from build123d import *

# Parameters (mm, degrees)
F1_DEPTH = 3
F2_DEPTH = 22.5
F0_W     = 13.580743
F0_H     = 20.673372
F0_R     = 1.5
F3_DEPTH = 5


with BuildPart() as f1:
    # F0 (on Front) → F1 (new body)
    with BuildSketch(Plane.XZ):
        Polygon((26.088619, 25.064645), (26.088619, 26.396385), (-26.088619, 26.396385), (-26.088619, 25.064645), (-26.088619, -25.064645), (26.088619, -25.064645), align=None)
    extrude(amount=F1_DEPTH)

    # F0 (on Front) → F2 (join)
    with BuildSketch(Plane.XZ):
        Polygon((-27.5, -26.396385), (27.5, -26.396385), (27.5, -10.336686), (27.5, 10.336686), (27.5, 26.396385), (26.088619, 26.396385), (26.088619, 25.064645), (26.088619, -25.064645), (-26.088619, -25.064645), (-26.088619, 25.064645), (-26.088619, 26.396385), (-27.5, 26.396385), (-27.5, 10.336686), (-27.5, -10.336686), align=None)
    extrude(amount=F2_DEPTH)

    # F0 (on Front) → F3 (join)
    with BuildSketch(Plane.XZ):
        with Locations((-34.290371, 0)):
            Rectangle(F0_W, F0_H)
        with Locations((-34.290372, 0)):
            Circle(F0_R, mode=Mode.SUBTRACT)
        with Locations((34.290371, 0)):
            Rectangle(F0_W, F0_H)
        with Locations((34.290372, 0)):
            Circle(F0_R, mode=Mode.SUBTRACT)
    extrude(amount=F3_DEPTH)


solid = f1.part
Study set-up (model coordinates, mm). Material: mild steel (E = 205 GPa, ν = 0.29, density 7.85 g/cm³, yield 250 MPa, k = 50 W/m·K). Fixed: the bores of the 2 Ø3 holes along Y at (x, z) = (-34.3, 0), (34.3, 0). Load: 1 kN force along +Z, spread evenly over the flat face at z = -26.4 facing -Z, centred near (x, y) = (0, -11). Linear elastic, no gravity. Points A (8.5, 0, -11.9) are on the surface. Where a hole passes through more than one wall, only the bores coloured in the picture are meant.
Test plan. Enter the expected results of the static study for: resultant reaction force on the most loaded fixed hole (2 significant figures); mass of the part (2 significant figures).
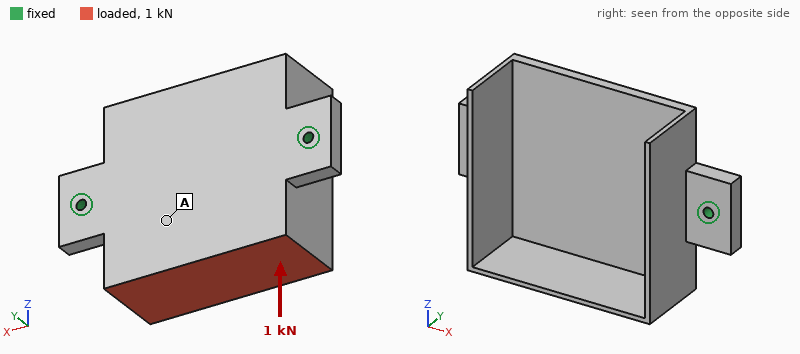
500 N
120 g
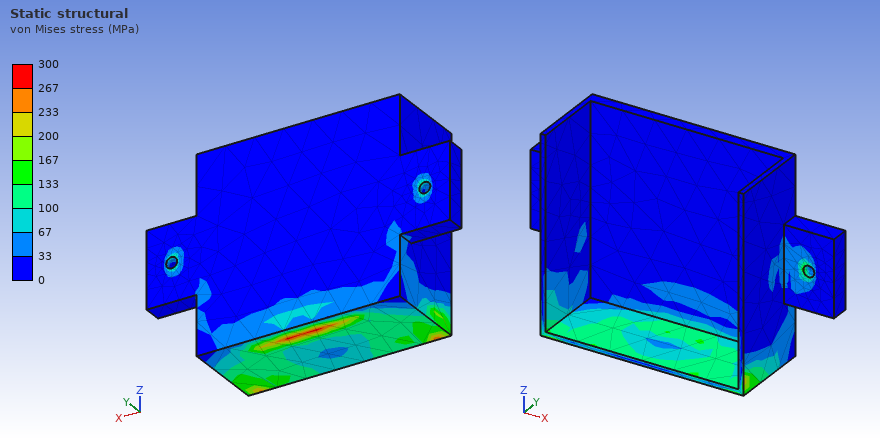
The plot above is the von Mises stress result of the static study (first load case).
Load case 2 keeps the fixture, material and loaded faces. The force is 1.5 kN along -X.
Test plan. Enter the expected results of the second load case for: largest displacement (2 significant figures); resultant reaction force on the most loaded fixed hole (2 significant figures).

47 µm
980 N
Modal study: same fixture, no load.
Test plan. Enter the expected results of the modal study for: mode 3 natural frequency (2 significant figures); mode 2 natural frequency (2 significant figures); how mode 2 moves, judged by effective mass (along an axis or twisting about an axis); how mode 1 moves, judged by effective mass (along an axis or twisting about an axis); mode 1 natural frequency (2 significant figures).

3500 Hz
3300 Hz
along Y
twisting about X
2700 Hz
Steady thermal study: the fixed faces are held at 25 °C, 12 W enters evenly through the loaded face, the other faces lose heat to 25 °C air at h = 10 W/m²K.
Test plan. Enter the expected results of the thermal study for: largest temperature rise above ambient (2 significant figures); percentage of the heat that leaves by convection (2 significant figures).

58 K
20 %
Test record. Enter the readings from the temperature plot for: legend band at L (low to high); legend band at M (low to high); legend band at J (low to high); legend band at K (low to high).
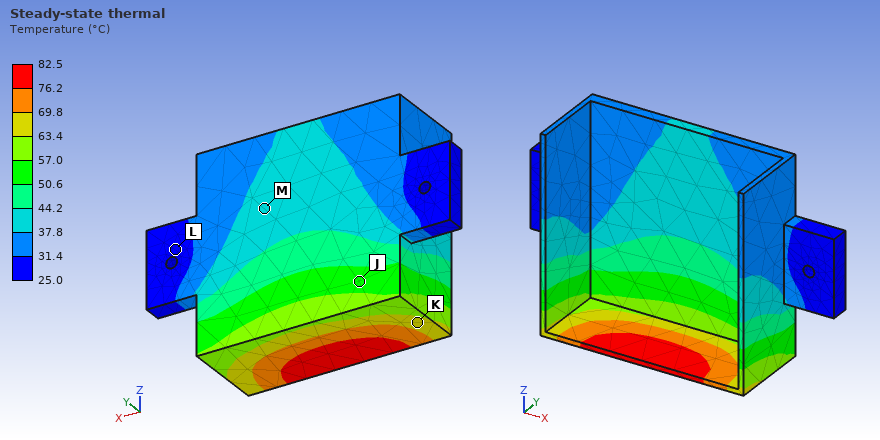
25.0 to 31.4 °C
37.8 to 44.2 °C
50.6 to 57.0 °C
63.4 to 69.8 °C
